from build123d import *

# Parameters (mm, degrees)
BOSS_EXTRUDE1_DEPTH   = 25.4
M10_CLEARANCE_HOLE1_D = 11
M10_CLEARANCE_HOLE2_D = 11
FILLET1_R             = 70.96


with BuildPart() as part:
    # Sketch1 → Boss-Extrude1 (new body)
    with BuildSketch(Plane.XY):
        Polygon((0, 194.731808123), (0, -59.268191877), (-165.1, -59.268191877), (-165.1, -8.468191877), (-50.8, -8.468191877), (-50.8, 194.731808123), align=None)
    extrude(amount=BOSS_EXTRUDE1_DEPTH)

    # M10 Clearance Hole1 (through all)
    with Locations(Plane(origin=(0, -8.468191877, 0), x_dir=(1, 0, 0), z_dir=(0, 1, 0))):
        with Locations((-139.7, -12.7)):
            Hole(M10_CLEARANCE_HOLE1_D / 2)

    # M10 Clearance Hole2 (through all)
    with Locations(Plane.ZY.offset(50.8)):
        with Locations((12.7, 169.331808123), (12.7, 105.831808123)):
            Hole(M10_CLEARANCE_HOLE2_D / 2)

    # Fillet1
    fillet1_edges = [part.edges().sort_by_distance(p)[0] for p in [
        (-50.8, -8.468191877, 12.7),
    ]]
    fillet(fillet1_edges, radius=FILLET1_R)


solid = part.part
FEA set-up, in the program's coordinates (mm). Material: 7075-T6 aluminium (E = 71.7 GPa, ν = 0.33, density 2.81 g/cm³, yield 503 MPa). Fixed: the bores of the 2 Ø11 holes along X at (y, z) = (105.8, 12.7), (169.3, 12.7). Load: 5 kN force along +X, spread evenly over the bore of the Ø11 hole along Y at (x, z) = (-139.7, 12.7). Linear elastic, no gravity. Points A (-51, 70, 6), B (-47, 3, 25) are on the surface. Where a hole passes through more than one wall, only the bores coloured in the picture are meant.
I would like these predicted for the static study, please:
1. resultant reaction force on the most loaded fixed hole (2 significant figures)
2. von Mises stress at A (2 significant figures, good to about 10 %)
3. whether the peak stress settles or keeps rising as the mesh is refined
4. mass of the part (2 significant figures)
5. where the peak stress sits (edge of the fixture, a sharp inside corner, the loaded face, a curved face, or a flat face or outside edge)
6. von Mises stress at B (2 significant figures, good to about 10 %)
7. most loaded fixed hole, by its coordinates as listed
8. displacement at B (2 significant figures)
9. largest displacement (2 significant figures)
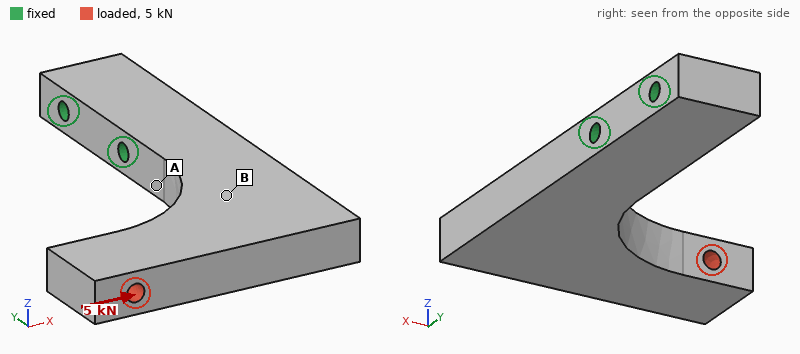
5.5 kN
48 MPa
keeps rising
1.4 kg
edge of the fixture
8.3 MPa
(105.8, 12.7)
0.15 mm
0.42 mm
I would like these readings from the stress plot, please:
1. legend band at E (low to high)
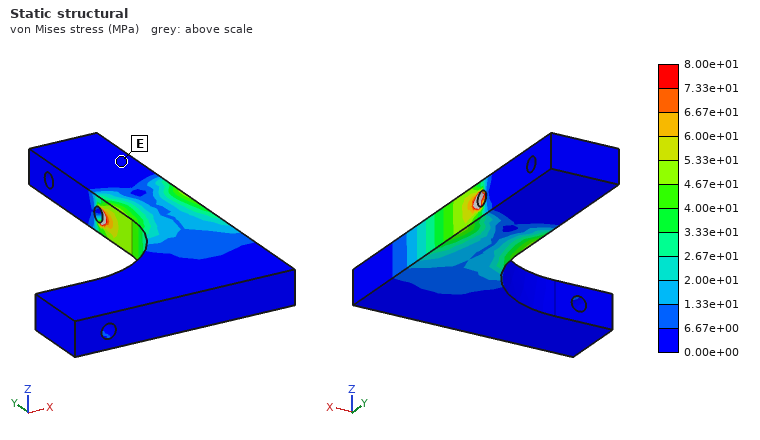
0.00e+00 to 6.67e+00 MPa
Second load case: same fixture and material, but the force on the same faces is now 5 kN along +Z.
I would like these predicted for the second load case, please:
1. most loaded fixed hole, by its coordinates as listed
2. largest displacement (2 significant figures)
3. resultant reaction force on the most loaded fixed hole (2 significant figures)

(105.8, 12.7)
3.0 mm
8.0 kN
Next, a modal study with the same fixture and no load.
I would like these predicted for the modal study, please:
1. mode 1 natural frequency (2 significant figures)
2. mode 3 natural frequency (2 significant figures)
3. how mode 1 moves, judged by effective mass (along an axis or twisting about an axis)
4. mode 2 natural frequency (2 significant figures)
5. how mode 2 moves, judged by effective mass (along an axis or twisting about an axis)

380 Hz
960 Hz
along Z
750 Hz
along X
